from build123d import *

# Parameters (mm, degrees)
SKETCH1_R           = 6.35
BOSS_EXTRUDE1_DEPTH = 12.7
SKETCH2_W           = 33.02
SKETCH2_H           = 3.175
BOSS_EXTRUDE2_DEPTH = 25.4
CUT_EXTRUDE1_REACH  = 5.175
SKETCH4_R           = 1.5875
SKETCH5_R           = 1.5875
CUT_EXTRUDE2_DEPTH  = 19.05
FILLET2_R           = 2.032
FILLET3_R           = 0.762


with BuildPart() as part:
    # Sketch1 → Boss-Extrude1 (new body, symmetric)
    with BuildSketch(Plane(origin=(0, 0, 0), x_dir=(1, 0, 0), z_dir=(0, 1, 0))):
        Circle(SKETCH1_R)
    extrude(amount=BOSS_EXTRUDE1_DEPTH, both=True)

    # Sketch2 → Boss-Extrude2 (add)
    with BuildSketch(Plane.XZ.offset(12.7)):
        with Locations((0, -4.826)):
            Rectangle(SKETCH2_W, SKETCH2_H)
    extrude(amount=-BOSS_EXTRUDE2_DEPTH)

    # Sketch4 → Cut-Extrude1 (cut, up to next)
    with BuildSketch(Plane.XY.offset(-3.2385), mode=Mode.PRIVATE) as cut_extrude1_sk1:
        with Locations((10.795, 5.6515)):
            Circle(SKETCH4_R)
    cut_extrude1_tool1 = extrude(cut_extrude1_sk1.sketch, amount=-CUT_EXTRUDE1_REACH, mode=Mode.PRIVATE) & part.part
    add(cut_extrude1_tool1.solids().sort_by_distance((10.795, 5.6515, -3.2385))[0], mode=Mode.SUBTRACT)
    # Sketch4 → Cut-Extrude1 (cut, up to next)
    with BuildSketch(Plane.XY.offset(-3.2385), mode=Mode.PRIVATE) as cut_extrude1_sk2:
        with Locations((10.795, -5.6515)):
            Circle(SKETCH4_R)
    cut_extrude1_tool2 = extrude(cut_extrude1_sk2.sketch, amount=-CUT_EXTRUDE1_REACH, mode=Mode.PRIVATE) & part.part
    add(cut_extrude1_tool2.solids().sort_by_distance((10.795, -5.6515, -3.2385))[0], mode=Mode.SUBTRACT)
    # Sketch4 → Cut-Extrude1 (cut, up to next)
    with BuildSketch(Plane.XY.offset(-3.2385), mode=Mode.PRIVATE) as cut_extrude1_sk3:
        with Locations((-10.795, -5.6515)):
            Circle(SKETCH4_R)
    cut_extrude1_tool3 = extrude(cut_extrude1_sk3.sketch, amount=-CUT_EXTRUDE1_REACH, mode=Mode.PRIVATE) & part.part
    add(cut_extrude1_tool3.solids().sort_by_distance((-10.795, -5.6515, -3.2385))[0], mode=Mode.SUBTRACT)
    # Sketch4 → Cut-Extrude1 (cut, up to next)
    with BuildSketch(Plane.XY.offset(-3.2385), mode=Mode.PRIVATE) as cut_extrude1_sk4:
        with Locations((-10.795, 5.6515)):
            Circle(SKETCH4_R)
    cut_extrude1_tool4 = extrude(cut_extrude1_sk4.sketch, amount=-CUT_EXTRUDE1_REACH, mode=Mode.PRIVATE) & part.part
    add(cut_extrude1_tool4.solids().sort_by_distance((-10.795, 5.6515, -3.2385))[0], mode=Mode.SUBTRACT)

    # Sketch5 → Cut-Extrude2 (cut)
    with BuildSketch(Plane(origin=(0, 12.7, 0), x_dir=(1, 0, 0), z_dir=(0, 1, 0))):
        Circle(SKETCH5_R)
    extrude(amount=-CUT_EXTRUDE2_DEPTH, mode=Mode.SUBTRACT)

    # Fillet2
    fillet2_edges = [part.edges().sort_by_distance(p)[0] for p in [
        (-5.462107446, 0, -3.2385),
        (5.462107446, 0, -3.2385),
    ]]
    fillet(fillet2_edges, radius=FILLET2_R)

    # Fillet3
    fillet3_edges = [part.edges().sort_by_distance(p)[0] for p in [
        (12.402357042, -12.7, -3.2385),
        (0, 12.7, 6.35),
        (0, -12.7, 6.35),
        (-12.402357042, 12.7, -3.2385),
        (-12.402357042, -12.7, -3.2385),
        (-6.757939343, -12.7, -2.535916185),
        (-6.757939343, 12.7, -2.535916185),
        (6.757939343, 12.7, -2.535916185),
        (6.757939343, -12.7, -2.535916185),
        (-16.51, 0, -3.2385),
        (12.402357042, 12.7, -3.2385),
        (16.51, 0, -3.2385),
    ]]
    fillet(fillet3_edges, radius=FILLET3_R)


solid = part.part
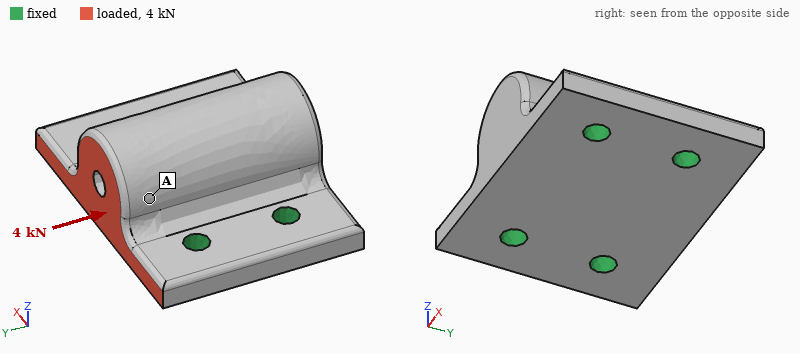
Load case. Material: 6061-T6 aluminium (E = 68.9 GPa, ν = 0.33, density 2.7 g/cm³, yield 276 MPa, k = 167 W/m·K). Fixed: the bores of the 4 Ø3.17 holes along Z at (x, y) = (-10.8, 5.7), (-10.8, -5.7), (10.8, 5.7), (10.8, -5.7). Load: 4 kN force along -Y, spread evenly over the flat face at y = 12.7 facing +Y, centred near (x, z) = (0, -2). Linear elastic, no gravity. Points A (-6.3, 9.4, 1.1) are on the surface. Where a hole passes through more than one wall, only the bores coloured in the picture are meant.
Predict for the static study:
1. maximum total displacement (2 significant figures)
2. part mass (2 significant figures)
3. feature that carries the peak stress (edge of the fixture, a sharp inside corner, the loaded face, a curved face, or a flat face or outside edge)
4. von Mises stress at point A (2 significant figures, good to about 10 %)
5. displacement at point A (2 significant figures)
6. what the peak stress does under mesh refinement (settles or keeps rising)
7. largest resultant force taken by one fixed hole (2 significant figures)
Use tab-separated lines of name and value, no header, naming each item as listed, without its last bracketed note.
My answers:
maximum total displacement	19 µm
part mass	14 g
feature that carries the peak stress	edge of the fixture
von Mises stress at point A	17 MPa
displacement at point A	13 µm
what the peak stress does under mesh refinement	keeps rising
largest resultant force taken by one fixed hole	1.3 kN
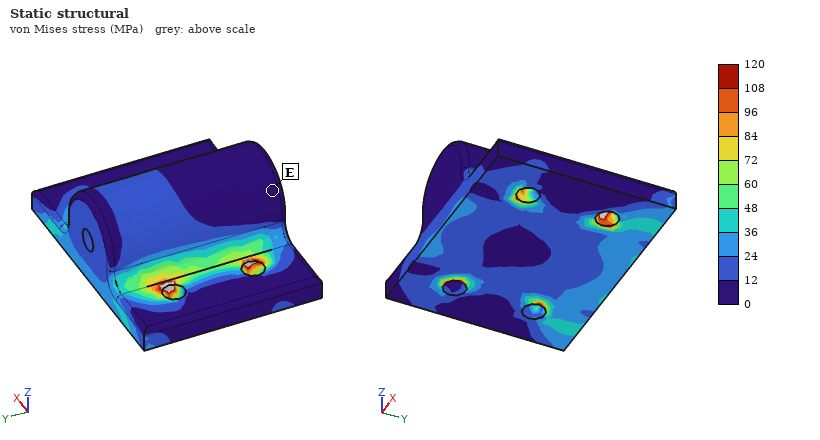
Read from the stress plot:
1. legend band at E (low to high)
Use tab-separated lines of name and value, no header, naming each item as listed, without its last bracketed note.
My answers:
legend band at E	0 to 12 MPa
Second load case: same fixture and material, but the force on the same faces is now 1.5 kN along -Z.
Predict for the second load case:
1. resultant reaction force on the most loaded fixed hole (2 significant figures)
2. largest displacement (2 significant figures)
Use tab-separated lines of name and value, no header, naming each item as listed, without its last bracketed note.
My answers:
resultant reaction force on the most loaded fixed hole	1.1 kN
largest displacement	25 µm
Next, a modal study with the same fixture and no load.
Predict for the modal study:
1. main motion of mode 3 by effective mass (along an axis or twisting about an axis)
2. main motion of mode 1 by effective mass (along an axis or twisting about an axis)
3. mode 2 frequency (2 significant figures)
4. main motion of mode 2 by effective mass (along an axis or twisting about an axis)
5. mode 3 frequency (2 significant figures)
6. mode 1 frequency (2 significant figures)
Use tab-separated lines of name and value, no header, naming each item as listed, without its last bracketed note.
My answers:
main motion of mode 3 by effective mass	along X
main motion of mode 1 by effective mass	along Y
mode 2 frequency	29 kHz
main motion of mode 2 by effective mass	along Z
mode 3 frequency	37 kHz
mode 1 frequency	20 kHz
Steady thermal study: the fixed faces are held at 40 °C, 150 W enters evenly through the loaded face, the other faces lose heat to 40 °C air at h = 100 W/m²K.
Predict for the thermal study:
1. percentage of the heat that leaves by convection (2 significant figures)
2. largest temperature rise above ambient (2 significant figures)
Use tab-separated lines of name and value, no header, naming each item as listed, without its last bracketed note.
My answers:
percentage of the heat that leaves by convection	3.3 %
largest temperature rise above ambient	68 K
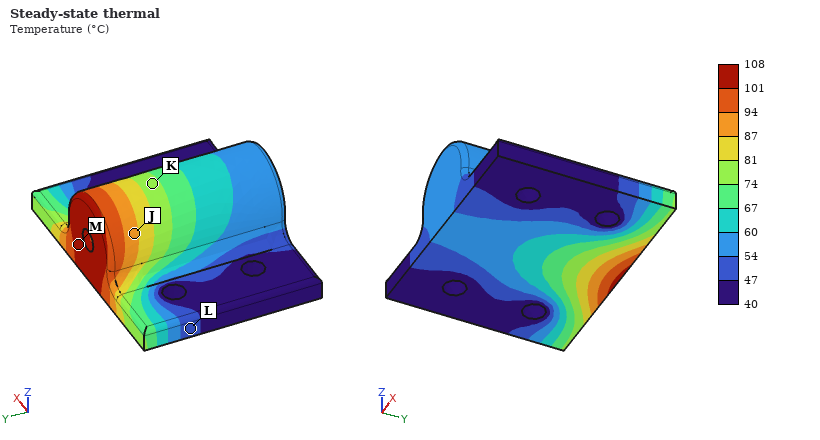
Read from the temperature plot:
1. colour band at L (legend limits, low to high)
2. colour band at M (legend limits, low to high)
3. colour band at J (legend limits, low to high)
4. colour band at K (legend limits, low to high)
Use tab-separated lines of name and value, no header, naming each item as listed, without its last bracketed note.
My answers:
colour band at L	47 to 54 °C
colour band at M	101 to 108 °C
colour band at J	87 to 94 °C
colour band at K	74 to 81 °C
